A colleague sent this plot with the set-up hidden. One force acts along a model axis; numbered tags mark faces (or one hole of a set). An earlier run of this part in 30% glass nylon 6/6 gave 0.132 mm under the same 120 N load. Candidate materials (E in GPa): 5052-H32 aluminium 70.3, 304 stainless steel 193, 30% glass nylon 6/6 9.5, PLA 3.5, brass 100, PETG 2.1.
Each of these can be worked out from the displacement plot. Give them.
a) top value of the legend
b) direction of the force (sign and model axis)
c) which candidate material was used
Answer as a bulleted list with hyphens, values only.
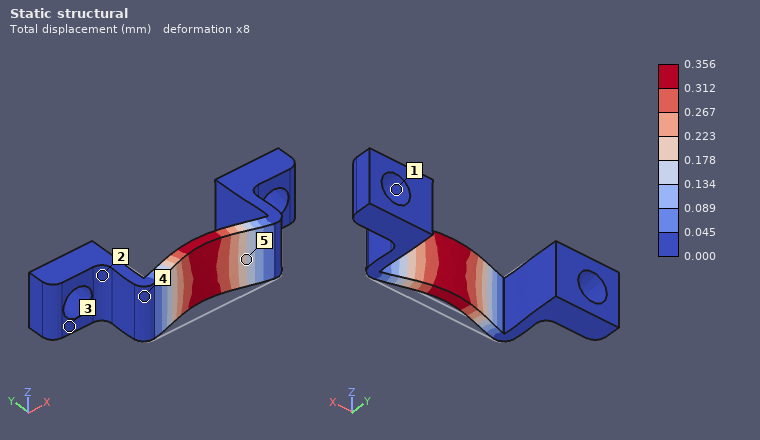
- 0.356 mm
- +Y
- PLA
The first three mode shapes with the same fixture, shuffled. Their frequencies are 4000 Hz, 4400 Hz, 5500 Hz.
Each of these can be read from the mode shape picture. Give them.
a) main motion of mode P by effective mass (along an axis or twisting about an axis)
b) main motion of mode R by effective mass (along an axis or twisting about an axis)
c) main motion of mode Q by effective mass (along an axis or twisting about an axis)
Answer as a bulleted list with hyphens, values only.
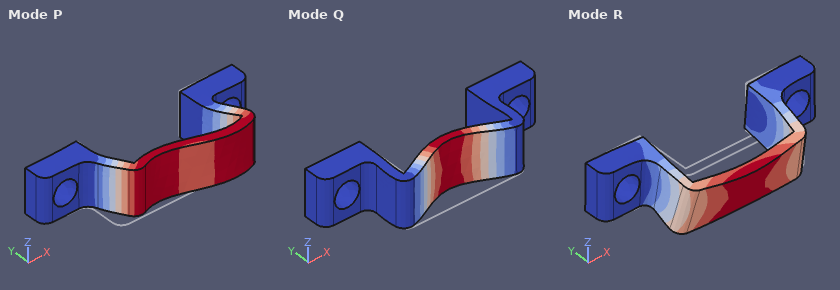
- along X
- along Z
- along Y
